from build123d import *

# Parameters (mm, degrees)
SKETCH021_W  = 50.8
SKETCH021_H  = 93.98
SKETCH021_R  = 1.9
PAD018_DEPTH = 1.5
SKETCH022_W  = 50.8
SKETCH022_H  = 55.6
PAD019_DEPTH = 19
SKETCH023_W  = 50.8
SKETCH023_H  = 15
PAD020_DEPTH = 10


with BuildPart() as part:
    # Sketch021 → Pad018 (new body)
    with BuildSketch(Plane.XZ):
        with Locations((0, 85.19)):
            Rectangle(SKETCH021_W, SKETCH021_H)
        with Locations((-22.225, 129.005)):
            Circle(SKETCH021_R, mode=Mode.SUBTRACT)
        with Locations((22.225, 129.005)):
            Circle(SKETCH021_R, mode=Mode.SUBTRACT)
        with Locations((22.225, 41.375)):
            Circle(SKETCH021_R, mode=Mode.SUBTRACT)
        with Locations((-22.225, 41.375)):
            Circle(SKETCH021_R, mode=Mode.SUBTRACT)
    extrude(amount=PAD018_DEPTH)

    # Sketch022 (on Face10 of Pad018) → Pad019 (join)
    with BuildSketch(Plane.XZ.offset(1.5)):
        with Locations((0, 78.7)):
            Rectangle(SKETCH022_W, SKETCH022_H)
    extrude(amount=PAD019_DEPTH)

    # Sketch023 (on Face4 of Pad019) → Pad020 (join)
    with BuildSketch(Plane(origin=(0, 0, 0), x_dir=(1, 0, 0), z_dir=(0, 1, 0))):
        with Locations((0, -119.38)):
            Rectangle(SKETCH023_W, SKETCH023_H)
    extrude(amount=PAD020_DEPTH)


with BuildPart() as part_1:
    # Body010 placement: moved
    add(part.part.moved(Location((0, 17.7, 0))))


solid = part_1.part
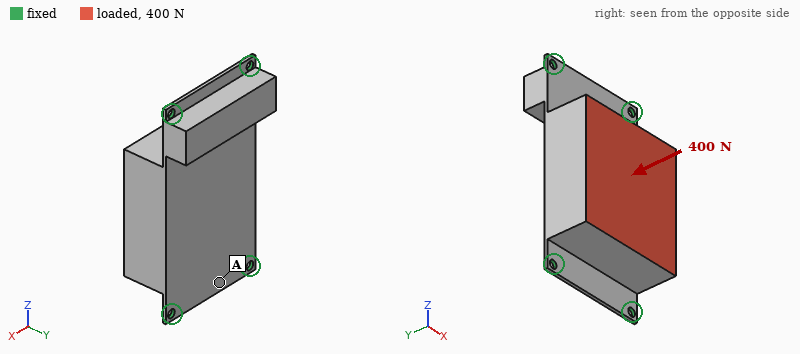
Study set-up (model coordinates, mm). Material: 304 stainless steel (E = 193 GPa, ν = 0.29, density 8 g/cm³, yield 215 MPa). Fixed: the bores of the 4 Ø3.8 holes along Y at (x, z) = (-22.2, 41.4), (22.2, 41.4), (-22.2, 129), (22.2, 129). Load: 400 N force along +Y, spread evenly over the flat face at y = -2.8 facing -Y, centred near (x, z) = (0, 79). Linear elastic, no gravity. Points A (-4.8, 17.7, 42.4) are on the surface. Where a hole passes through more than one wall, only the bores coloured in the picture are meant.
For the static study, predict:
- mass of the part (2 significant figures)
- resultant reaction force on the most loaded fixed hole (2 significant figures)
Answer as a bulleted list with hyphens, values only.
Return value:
- 550 g
- 140 N
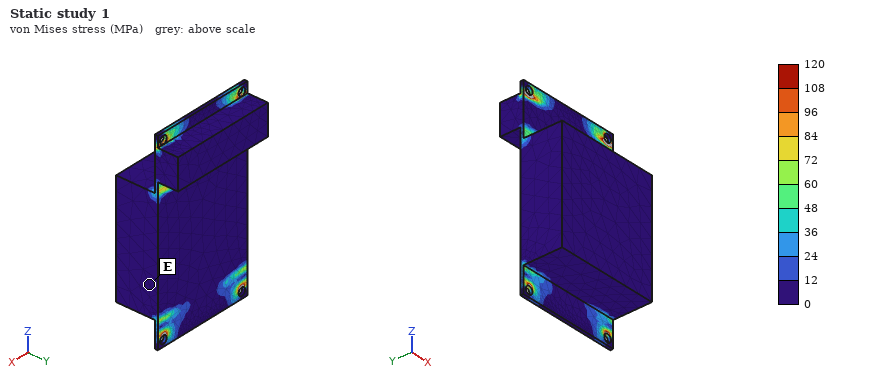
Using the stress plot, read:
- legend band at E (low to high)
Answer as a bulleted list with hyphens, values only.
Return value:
- 0 to 12 MPa
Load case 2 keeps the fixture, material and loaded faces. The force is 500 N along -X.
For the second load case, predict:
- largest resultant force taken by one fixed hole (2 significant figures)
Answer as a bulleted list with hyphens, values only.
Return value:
- 230 N
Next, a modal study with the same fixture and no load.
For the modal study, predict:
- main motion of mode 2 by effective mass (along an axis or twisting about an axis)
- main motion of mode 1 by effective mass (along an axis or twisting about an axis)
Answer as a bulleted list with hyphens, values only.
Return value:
- along X
- along Y
